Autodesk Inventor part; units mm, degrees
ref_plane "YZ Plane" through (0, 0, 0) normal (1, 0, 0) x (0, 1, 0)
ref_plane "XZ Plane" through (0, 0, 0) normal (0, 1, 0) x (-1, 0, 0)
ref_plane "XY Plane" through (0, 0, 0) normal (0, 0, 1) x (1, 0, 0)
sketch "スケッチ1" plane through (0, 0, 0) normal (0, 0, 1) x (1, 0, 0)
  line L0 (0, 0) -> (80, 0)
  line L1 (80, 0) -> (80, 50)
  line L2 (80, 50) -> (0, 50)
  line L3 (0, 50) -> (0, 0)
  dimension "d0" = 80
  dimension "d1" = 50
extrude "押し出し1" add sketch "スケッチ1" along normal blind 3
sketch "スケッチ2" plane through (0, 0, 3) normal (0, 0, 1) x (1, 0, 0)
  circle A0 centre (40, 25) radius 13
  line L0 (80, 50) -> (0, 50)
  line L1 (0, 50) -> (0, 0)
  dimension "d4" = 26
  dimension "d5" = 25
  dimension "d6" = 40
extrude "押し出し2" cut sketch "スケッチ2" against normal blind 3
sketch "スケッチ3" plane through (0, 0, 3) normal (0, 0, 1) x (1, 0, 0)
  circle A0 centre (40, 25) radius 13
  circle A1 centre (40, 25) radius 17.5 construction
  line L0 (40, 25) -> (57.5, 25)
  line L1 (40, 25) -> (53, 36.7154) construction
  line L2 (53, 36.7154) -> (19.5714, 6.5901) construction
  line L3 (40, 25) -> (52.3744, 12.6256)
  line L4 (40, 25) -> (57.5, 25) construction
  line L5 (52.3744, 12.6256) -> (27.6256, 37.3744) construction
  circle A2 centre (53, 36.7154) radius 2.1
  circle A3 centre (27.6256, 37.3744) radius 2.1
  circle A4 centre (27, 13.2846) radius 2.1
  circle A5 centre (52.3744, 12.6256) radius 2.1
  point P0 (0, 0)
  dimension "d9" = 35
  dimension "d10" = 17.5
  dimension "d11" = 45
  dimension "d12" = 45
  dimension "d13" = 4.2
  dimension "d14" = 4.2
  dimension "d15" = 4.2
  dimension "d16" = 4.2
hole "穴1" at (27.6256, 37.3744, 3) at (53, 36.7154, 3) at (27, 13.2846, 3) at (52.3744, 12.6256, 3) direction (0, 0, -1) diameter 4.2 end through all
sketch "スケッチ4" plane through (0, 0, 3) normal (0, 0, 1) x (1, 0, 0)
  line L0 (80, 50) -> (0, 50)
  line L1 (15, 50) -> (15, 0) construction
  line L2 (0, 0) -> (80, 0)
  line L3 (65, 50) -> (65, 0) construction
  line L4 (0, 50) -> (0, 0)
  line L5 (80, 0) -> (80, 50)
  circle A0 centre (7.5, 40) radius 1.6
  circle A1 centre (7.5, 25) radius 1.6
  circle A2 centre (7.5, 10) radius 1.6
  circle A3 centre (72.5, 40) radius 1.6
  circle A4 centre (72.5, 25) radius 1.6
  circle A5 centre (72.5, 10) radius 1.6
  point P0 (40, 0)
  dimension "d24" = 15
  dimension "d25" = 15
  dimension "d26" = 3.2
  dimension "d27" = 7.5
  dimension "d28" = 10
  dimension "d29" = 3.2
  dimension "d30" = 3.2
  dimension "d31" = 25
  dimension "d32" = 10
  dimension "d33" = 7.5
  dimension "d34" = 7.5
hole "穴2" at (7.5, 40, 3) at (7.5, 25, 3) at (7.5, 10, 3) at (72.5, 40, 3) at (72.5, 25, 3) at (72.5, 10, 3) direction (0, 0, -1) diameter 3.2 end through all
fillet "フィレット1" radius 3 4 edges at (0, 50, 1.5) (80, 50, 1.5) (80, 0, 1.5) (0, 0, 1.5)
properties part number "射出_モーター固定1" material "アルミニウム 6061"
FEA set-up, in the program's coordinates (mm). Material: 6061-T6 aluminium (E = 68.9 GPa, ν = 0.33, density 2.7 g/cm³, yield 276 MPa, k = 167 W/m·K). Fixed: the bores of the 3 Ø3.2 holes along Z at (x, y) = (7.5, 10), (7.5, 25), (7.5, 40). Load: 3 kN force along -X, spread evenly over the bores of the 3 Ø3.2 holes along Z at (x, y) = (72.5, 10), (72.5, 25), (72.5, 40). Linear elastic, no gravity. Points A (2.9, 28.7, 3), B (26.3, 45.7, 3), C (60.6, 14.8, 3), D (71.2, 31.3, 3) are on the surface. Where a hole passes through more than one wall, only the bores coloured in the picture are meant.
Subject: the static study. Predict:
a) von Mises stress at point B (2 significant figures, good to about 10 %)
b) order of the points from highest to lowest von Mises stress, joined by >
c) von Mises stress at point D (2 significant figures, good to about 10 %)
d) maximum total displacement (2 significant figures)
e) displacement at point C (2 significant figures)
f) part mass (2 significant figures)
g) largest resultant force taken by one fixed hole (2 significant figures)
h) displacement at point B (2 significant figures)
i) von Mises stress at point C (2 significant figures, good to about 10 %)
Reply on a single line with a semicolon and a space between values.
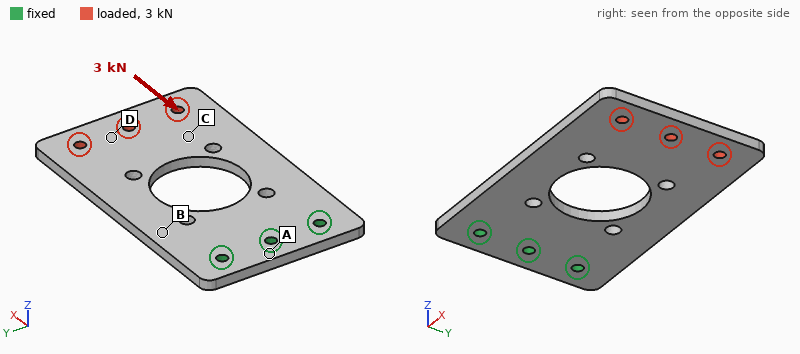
36 MPa; B > C > D > A; 14 MPa; 44 µm; 37 µm; 27 g; 1.3 kN; 15 µm; 24 MPa
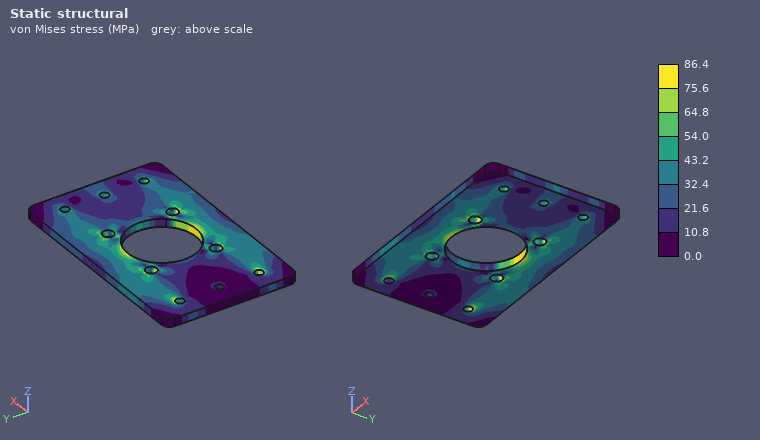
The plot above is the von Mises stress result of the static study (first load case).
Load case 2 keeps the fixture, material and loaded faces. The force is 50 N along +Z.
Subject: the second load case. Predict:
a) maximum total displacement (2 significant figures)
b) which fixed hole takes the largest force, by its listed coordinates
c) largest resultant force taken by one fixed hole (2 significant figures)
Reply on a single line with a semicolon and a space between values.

0.96 mm; (7.5, 25); 36 N
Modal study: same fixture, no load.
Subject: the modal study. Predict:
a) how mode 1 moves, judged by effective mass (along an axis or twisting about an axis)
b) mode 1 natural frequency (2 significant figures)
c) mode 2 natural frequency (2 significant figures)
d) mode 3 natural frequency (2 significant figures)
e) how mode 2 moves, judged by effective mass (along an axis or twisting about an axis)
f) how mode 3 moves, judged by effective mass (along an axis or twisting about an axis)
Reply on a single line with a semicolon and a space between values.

along Z; 420 Hz; 1300 Hz; 2800 Hz; twisting about X; along Z
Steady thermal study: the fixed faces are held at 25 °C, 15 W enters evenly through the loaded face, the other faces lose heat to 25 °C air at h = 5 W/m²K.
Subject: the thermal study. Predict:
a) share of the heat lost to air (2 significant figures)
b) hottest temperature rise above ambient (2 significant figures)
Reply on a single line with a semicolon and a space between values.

7.4 %; 58 K
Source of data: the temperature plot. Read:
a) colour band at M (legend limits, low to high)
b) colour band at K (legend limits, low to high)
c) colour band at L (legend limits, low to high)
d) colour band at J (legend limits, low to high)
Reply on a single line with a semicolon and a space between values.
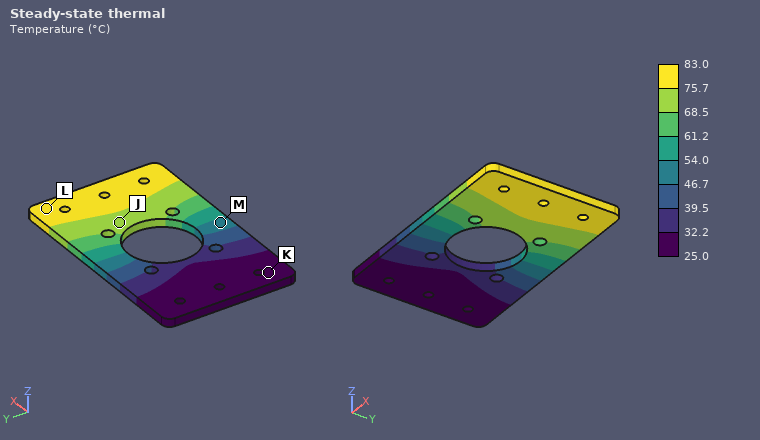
46.7 to 54.0 °C; 25.0 to 32.2 °C; 75.7 to 83.0 °C; 68.5 to 75.7 °C
